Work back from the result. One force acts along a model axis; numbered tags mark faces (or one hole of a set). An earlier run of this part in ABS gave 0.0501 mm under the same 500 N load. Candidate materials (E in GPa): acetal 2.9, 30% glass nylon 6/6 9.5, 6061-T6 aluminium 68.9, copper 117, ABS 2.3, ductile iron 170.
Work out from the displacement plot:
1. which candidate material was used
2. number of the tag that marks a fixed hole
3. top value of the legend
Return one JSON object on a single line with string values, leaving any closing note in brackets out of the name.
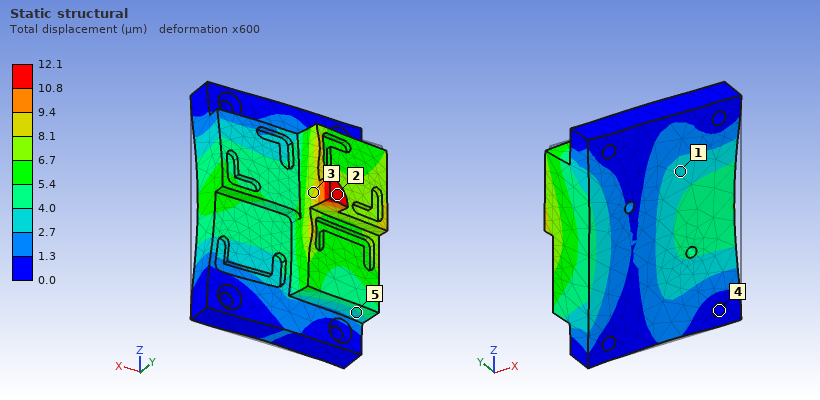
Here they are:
{"which candidate material was used": "30% glass nylon 6/6", "number of the tag that marks a fixed hole": "4", "top value of the legend": "12.1 µm"}
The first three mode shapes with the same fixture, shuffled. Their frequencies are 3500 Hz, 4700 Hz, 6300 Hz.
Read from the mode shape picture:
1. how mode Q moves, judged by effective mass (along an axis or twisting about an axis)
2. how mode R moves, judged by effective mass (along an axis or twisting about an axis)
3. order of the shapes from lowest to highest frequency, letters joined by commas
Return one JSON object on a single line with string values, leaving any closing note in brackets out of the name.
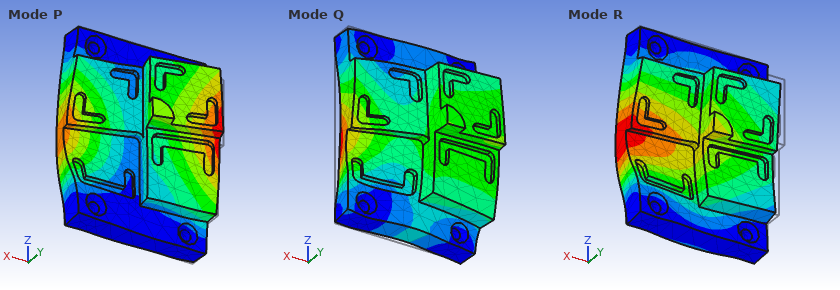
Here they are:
{"how mode Q moves, judged by effective mass": "along X", "how mode R moves, judged by effective mass": "along Y", "order of the shapes from lowest to highest frequency, letters joined by commas": "R, P, Q"}
